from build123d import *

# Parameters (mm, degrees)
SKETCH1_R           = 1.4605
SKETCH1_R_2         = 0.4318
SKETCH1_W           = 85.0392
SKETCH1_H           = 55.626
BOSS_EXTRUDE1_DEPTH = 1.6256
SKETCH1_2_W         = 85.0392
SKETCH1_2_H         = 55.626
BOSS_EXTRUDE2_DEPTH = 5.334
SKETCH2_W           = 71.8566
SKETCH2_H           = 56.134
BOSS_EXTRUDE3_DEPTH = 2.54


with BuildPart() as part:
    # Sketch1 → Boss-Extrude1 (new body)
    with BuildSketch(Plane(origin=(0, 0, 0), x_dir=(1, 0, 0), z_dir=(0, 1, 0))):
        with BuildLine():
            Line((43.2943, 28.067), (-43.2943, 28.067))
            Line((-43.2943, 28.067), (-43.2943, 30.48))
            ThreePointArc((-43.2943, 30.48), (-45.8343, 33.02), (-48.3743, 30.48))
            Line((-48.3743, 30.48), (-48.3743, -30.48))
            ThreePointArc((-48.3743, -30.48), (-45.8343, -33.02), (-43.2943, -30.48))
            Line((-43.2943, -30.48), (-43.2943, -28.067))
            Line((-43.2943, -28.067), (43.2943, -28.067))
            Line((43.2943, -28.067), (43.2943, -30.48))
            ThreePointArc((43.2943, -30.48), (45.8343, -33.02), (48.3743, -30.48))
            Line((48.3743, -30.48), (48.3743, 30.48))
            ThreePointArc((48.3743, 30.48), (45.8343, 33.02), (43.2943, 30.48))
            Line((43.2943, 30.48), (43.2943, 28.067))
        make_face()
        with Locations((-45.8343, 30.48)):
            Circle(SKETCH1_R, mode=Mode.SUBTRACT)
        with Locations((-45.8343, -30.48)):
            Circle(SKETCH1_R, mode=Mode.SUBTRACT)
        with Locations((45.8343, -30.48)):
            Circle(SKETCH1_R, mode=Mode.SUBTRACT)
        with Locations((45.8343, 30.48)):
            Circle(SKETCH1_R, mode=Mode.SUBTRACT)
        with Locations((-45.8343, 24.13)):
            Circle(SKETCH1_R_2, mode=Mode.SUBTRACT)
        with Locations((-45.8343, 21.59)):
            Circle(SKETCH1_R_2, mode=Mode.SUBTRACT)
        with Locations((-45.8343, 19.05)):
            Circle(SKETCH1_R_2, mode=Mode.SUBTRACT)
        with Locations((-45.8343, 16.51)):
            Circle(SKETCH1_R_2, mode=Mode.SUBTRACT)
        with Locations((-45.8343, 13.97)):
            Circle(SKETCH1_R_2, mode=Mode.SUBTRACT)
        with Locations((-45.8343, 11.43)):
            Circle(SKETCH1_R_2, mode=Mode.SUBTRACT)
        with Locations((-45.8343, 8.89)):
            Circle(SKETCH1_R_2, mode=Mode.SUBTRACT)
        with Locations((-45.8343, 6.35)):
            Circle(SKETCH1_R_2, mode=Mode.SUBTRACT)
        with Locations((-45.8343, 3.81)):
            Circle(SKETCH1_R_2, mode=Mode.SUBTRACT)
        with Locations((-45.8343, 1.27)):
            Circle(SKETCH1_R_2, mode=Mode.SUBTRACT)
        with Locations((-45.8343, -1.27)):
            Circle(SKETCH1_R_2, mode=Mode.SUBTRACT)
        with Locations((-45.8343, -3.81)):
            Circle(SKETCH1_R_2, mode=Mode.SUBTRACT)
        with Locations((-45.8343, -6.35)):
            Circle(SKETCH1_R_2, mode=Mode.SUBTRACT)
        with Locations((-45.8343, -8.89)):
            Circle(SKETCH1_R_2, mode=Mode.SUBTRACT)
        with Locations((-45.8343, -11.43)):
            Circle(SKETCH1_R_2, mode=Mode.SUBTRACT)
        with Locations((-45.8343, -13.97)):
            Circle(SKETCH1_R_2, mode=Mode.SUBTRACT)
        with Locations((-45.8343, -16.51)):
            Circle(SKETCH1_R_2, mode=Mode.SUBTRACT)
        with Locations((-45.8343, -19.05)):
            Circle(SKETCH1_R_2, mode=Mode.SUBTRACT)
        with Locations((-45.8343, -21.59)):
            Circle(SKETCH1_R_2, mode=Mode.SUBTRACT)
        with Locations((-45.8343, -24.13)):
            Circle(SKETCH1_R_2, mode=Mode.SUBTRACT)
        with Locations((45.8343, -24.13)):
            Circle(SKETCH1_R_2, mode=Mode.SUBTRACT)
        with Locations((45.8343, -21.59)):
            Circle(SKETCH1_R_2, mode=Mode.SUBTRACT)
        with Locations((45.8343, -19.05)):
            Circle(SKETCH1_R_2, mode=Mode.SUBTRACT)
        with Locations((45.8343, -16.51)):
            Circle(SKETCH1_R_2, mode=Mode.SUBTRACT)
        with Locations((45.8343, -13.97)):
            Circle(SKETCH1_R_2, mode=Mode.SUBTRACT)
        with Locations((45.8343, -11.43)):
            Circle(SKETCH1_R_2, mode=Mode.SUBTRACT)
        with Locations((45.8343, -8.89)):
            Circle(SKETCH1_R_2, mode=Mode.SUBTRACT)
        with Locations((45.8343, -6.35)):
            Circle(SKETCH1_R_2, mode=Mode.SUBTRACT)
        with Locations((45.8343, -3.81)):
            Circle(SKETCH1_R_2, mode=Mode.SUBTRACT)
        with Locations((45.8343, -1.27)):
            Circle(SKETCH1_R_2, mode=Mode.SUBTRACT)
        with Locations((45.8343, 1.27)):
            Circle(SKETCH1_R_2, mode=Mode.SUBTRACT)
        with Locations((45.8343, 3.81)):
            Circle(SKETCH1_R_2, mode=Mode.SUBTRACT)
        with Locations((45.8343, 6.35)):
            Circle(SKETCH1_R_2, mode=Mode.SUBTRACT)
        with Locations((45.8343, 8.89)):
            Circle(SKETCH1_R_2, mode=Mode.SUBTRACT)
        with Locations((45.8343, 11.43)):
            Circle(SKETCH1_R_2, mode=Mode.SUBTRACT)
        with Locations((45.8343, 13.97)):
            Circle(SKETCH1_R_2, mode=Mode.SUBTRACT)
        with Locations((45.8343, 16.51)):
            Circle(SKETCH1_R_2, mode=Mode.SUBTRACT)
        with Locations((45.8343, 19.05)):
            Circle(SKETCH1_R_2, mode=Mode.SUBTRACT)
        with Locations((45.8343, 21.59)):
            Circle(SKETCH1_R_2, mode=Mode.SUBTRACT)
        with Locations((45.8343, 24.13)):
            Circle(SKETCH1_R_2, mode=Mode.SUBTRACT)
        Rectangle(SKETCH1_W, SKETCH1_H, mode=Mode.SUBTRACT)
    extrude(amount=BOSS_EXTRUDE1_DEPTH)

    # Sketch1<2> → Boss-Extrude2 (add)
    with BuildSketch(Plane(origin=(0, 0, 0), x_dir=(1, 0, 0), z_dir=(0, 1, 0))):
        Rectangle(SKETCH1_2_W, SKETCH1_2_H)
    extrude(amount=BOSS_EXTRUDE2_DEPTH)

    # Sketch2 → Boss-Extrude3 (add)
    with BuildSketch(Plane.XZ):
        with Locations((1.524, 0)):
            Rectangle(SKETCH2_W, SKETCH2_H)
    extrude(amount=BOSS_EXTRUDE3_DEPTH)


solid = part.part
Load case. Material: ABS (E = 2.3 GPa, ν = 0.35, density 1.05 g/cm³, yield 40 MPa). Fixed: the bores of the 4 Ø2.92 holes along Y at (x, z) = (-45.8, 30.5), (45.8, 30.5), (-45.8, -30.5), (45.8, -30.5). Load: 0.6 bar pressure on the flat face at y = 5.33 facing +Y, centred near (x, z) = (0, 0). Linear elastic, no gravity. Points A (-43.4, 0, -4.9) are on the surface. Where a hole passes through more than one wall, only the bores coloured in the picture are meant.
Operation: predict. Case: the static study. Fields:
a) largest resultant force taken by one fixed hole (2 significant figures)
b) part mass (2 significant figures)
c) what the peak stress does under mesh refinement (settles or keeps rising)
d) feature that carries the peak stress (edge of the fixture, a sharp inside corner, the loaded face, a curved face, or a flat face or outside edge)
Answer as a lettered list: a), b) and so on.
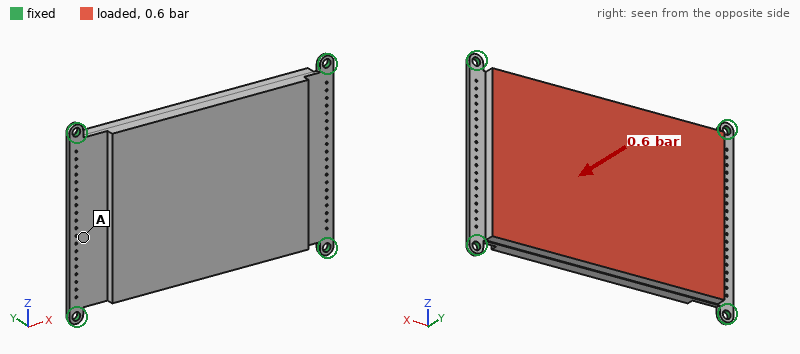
a) 93 N
b) 39 g
c) keeps rising
d) edge of the fixture
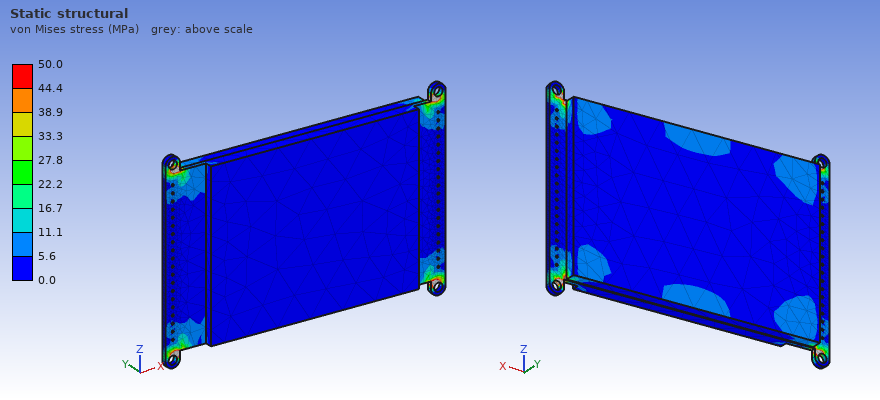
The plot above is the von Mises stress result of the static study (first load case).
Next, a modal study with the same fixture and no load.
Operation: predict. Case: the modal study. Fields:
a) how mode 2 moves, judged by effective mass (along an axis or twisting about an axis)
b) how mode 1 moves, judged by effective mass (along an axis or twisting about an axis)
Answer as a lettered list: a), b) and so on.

a) twisting about X
b) along Y
